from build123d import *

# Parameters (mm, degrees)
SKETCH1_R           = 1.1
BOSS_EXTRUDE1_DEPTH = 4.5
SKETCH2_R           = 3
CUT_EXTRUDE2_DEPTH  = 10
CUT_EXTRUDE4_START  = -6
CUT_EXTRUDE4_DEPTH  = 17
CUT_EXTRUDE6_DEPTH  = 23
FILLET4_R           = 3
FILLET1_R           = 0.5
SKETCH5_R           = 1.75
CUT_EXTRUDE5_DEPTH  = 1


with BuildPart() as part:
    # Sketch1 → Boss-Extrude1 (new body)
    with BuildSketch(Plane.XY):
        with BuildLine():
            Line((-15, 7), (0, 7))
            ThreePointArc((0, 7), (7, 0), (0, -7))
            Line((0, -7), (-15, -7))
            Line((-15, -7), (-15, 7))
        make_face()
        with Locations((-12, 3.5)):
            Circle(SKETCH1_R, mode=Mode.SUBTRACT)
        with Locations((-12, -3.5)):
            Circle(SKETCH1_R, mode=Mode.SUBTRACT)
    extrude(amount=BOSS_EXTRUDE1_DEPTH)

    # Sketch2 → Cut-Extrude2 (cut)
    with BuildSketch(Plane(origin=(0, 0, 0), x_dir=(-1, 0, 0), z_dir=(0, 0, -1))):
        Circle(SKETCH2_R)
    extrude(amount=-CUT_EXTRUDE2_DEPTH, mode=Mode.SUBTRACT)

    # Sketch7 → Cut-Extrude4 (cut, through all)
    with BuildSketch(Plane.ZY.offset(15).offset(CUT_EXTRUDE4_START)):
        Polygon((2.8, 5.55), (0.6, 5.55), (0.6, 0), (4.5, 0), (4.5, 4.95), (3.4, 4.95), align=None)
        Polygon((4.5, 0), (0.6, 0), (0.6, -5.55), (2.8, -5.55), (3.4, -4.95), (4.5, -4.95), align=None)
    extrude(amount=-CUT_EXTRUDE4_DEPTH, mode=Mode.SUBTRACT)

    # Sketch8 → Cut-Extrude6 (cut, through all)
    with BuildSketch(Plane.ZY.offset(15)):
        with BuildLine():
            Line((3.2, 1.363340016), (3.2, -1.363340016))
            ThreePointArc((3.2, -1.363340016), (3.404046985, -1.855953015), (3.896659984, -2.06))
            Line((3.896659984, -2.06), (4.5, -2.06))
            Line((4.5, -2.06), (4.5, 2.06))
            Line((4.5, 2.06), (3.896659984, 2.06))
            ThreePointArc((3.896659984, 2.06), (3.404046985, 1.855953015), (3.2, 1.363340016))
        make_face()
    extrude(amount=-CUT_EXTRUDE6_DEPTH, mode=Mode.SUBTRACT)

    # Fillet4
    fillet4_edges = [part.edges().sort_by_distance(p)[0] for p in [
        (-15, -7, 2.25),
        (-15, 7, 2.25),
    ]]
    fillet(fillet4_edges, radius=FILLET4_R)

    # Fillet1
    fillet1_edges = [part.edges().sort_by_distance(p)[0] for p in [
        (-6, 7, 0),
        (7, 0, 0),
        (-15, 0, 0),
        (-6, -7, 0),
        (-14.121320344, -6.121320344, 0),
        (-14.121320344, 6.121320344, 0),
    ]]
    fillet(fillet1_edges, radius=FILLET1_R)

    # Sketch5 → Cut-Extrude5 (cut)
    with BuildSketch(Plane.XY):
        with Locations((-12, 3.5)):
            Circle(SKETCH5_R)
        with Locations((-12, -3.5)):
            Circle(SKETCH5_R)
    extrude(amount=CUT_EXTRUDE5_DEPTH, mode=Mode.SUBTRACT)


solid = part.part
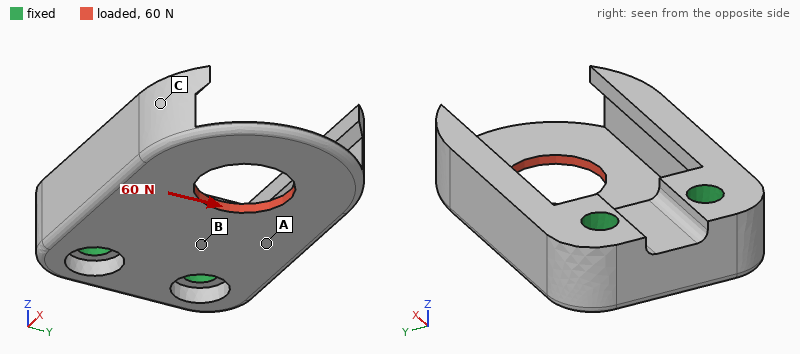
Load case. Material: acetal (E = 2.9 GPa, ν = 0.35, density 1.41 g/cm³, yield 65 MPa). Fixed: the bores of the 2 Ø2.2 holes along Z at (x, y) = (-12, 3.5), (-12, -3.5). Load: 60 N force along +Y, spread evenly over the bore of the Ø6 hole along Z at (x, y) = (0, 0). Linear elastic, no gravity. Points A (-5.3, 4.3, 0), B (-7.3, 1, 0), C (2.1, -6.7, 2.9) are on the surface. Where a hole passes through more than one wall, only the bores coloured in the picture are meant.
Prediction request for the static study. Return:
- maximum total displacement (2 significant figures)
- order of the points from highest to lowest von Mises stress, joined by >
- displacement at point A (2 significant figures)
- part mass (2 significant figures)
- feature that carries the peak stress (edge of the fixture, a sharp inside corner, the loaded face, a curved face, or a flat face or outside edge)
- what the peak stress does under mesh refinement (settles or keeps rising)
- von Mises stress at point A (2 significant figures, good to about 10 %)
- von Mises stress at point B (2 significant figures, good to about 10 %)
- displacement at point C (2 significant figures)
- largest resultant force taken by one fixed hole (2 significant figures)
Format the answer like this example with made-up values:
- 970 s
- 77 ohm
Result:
- 0.28 mm
- B > A > C
- 0.069 mm
- 0.77 g
- a sharp inside corner
- keeps rising
- 9.2 MPa
- 16 MPa
- 0.22 mm
- 77 N
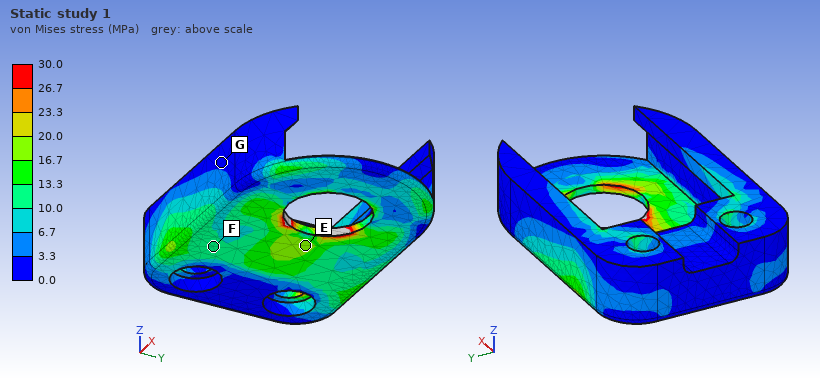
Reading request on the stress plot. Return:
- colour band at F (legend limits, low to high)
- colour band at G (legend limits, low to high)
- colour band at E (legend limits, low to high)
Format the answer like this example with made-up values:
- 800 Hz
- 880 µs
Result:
- 10.0 to 13.3 MPa
- 0.0 to 3.3 MPa
- 16.7 to 20.0 MPa
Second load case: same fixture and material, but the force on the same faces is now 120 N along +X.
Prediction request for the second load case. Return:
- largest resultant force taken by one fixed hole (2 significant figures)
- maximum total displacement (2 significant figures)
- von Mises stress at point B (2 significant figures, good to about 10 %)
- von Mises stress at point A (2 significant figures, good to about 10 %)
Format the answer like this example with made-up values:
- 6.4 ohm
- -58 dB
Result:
- 60 N
- 0.24 mm
- 12 MPa
- 15 MPa
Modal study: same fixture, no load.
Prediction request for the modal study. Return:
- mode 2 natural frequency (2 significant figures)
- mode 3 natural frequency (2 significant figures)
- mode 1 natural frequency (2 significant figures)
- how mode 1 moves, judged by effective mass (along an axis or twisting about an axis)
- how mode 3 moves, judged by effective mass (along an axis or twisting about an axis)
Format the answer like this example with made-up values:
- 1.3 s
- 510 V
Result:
- 4100 Hz
- 5700 Hz
- 3200 Hz
- along Z
- along Y
